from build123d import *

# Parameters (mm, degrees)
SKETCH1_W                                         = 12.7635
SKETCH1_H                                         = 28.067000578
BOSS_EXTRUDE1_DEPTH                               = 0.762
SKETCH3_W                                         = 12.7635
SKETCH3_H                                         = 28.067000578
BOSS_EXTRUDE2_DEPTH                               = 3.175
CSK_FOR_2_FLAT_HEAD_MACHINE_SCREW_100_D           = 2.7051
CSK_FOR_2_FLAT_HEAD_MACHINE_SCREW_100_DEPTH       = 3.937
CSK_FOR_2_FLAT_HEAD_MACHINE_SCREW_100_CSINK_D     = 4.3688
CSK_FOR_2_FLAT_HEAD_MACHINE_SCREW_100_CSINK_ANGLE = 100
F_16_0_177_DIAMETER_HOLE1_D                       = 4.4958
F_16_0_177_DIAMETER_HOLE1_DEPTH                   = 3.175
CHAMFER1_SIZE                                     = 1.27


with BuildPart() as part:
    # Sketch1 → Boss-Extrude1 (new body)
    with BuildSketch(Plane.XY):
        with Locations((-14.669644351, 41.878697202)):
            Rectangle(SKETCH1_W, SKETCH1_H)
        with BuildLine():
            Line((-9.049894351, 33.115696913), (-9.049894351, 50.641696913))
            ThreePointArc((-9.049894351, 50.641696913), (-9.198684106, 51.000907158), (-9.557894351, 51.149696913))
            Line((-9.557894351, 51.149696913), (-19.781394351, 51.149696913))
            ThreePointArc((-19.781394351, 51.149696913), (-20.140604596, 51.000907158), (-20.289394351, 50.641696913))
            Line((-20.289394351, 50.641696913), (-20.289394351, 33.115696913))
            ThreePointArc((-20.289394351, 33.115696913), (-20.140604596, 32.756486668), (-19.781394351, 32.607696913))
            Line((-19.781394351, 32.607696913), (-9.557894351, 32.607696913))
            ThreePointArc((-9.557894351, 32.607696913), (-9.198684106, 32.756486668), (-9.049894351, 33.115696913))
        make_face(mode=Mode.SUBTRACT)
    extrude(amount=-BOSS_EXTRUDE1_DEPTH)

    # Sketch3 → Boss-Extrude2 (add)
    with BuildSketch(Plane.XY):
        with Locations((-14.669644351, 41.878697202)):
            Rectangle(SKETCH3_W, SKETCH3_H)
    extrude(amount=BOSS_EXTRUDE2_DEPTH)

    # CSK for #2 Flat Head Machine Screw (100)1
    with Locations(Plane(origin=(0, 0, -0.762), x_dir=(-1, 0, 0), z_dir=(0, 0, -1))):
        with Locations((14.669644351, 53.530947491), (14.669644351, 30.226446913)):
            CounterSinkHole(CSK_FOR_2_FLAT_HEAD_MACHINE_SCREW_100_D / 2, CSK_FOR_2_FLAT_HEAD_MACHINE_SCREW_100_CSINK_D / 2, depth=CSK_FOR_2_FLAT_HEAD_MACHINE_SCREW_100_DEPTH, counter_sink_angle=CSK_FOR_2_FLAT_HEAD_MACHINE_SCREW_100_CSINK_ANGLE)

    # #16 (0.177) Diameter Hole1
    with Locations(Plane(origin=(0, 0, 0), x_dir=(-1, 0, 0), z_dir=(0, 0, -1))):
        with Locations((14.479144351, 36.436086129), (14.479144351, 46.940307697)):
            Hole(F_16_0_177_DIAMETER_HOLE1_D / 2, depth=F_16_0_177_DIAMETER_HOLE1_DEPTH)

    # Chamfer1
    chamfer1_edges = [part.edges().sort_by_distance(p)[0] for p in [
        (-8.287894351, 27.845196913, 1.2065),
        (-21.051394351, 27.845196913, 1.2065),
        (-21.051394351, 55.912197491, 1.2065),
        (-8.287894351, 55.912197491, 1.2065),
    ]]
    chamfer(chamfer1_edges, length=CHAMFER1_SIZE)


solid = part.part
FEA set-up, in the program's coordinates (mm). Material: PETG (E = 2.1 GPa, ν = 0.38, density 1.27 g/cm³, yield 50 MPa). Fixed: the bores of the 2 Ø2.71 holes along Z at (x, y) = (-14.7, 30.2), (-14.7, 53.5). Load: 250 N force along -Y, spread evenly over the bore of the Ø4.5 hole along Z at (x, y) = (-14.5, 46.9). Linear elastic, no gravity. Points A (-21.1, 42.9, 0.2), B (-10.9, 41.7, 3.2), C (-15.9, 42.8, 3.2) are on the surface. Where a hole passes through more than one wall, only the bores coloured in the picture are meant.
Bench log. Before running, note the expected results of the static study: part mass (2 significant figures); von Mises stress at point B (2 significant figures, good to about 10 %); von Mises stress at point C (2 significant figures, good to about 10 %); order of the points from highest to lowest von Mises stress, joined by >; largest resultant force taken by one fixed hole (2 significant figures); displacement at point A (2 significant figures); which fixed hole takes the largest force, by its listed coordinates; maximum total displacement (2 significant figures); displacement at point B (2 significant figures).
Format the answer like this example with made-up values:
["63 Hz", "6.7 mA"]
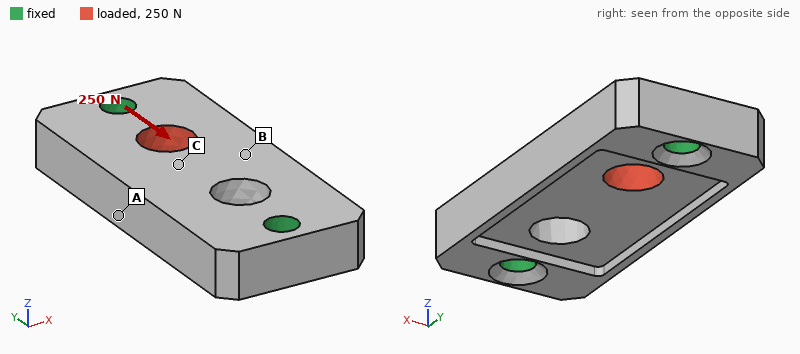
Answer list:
["1.4 g", "3.1 MPa", "4.5 MPa", "C > B > A", "170 N", "16 µm", "(-14.7, 53.5)", "36 µm", "22 µm"]
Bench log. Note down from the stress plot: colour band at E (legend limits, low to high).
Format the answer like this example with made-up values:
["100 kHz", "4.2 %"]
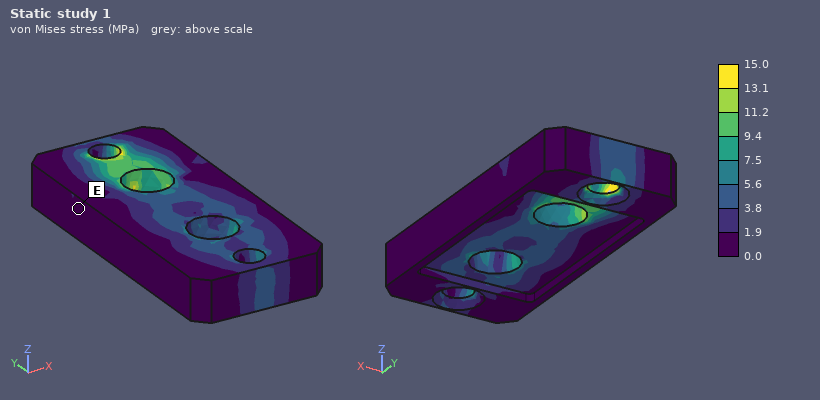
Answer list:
["0.0 to 1.9 MPa"]
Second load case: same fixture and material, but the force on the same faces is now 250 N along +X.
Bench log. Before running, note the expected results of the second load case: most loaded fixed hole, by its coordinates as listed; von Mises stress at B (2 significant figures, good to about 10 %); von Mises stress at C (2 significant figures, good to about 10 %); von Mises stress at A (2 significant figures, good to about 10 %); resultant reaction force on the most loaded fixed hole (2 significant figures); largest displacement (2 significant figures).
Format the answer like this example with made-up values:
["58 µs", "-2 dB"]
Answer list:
["(-14.7, 53.5)", "3.5 MPa", "3.6 MPa", "10 MPa", "180 N", "83 µm"]
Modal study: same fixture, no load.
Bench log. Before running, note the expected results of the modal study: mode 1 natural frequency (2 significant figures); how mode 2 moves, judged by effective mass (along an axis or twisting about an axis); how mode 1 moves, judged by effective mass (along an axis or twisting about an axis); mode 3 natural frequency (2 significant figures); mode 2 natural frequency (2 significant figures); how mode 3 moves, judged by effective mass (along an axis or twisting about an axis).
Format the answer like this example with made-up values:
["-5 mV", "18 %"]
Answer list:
["6700 Hz", "twisting about Y", "along Z", "11 kHz", "7500 Hz", "along X"]
